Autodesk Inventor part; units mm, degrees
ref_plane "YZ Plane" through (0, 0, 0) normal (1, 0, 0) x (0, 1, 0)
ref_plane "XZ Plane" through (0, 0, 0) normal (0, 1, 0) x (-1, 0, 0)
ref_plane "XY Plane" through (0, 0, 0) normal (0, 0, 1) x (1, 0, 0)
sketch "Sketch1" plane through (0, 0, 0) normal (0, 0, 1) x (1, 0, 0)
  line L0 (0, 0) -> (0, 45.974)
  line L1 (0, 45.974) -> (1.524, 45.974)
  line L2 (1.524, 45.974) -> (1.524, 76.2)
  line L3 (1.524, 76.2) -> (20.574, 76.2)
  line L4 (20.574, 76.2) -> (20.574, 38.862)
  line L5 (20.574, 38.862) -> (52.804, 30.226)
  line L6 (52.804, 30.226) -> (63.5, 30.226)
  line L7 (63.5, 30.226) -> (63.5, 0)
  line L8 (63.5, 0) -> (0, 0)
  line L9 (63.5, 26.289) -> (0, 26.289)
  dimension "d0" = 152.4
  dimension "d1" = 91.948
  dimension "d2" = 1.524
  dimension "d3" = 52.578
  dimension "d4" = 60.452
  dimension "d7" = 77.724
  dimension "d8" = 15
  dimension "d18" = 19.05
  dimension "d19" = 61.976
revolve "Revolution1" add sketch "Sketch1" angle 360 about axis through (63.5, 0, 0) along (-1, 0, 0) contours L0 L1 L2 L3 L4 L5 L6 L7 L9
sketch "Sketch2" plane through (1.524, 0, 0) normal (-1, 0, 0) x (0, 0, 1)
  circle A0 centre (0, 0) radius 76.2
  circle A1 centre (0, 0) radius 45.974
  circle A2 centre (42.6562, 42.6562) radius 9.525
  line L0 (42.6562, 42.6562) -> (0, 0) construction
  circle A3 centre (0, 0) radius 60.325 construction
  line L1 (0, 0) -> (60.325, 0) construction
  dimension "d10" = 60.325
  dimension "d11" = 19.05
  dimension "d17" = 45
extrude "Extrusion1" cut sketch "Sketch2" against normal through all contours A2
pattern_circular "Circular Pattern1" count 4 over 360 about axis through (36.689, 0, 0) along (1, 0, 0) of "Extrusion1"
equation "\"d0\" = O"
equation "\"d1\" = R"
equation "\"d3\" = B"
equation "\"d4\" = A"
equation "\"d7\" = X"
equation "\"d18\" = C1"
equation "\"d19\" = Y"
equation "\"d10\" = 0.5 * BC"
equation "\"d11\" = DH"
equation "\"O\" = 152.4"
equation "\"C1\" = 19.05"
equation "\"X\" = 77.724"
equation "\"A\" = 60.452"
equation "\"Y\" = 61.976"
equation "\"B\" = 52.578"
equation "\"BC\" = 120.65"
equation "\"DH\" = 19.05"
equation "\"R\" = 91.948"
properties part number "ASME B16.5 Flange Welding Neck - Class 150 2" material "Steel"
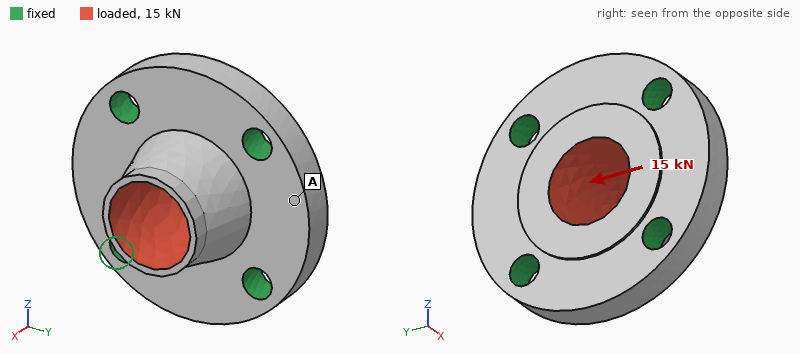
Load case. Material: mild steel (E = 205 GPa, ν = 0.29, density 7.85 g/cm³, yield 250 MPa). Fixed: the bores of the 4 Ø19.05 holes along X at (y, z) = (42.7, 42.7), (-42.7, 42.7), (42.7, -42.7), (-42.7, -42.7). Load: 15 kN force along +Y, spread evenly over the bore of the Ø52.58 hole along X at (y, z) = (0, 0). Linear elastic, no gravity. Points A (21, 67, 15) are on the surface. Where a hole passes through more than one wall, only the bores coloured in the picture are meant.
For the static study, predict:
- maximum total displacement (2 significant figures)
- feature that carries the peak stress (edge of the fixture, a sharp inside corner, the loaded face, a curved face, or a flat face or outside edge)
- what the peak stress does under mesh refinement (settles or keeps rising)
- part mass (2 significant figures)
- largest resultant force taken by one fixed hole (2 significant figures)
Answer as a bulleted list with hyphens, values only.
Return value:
- 7.8 µm
- edge of the fixture
- keeps rising
- 2.7 kg
- 4.3 kN
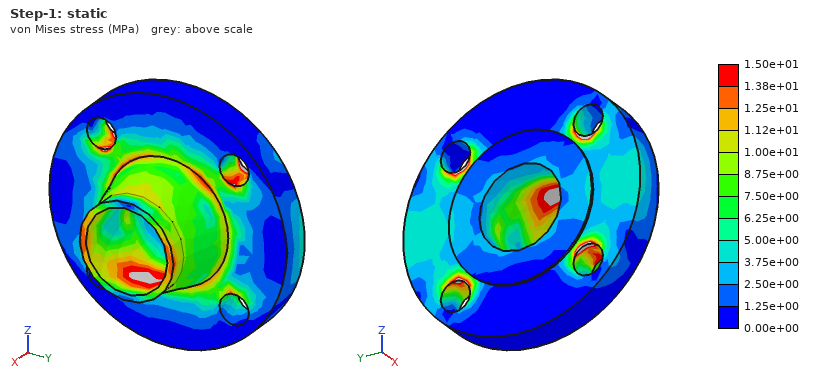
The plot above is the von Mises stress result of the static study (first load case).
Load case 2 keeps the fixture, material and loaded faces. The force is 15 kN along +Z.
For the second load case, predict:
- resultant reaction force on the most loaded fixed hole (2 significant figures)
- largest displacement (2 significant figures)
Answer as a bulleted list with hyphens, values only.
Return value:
- 4.3 kN
- 7.8 µm
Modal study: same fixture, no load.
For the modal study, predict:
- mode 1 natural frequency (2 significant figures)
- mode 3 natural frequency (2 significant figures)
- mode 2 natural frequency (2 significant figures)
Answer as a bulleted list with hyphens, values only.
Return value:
- 9400 Hz
- 10 kHz
- 10 kHz
